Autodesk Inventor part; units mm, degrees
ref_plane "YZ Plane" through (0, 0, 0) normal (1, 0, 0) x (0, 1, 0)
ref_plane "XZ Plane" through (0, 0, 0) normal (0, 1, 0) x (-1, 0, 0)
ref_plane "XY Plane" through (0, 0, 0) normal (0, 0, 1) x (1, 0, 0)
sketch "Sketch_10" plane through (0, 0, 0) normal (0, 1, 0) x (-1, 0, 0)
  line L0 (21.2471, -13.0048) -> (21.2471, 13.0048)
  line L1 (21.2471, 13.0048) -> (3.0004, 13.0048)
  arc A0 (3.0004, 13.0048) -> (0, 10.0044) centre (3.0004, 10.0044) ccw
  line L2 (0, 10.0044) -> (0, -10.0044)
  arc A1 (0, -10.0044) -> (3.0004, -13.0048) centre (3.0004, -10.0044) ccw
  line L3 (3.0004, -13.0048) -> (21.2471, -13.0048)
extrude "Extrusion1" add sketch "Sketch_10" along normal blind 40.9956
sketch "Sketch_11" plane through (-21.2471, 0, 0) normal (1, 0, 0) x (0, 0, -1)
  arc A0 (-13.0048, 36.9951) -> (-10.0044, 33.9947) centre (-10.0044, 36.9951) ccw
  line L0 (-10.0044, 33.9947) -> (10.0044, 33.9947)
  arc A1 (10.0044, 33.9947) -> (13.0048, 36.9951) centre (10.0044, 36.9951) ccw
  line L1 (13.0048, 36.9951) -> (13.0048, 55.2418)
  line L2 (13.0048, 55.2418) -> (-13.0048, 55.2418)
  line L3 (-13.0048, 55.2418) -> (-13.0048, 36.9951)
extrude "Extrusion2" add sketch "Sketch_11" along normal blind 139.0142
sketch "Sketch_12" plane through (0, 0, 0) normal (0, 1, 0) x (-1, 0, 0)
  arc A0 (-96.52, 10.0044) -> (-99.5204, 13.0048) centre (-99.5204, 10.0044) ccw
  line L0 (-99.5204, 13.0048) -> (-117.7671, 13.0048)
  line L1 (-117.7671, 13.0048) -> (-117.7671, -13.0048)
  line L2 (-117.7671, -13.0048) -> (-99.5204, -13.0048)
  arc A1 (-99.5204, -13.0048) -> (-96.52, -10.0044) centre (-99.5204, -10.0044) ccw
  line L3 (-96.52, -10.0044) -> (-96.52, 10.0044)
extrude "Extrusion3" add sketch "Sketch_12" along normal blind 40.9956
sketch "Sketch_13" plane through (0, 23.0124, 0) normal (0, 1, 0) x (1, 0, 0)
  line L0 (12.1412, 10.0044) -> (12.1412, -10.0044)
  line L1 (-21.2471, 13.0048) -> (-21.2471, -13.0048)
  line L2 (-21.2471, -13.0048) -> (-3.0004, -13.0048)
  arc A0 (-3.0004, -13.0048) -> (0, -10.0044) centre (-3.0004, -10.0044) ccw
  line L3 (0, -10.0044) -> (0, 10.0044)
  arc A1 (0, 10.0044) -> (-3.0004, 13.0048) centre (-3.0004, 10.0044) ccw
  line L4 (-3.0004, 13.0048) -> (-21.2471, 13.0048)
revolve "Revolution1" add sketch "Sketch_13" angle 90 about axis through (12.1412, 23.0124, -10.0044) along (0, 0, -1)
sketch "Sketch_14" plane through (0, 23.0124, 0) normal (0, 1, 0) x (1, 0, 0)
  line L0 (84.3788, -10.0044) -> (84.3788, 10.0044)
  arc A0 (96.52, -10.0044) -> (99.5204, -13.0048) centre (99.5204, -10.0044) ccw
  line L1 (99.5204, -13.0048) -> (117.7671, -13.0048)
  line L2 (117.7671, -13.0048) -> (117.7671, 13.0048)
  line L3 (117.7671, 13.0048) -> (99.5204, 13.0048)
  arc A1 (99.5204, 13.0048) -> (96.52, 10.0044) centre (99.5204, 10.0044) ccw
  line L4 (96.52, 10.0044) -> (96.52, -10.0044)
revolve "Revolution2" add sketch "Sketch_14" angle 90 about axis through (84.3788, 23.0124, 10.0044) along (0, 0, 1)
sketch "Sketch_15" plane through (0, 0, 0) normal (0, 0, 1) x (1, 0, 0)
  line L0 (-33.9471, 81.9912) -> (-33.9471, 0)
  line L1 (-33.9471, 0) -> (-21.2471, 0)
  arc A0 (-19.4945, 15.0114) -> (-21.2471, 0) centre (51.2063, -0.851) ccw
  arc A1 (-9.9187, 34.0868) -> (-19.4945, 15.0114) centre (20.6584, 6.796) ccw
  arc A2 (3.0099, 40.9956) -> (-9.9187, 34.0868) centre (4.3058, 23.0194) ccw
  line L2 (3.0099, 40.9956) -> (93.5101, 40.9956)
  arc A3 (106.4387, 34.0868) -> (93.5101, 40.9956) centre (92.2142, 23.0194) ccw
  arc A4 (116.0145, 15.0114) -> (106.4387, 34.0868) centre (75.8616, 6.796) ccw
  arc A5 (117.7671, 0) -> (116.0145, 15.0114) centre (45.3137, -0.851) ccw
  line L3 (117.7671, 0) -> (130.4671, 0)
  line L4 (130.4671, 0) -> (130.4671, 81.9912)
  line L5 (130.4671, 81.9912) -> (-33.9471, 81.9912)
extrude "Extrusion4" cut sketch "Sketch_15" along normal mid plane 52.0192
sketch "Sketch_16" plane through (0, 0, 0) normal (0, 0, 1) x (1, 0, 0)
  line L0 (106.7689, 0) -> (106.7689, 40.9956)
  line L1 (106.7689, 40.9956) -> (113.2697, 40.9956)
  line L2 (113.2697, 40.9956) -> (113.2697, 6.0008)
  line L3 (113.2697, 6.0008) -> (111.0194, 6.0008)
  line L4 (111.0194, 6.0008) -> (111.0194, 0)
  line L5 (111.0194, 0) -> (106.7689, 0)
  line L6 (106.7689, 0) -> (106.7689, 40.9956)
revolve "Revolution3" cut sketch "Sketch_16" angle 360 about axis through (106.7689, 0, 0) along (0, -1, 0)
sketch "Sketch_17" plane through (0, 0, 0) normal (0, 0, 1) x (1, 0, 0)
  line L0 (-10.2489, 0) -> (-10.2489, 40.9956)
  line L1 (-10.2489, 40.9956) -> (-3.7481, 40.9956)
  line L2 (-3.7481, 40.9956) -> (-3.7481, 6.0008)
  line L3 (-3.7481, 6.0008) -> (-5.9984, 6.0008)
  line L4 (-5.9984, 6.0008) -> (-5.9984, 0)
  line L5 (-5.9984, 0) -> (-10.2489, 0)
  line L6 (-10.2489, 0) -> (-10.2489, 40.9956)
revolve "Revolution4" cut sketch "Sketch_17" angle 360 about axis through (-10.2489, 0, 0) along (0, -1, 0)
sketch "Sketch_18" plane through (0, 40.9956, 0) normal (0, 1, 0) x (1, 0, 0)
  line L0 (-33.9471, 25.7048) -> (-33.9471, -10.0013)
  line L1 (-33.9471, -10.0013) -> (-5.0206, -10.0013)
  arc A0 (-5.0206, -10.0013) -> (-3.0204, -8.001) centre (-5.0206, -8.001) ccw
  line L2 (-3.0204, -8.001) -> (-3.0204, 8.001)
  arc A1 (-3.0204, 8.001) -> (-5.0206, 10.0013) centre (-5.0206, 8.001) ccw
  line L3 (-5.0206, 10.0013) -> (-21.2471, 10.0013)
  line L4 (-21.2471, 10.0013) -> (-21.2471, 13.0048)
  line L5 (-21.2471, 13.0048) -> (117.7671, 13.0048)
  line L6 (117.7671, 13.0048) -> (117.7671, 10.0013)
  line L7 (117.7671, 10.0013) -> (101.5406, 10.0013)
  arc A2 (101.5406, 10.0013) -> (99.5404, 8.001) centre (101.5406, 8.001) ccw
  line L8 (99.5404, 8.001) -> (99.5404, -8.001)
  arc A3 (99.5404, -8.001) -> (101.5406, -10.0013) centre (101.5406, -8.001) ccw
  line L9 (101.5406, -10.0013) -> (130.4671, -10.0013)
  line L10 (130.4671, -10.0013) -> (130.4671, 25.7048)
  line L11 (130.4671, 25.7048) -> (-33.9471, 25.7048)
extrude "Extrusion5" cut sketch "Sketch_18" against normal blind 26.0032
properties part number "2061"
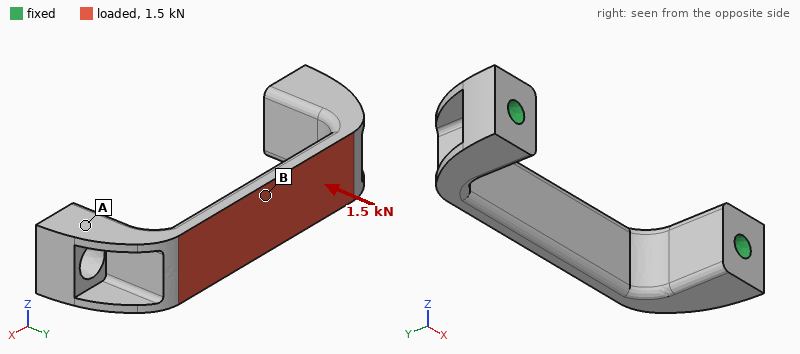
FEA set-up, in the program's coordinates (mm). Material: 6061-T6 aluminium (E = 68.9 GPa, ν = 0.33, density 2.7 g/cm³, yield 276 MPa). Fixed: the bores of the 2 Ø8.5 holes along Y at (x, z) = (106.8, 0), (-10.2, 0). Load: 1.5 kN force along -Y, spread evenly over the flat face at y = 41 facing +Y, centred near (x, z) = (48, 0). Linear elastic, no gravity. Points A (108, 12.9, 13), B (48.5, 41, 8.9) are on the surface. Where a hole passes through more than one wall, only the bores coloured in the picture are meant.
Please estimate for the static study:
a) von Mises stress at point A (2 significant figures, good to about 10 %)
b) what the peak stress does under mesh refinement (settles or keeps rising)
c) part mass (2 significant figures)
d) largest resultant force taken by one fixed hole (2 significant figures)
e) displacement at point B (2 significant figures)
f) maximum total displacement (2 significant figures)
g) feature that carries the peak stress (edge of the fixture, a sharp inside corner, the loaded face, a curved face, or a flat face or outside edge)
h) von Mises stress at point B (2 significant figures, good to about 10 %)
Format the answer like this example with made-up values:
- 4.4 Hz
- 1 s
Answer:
- 6.2 MPa
- keeps rising
- 100 g
- 990 N
- 0.10 mm
- 0.10 mm
- a sharp inside corner
- 38 MPa
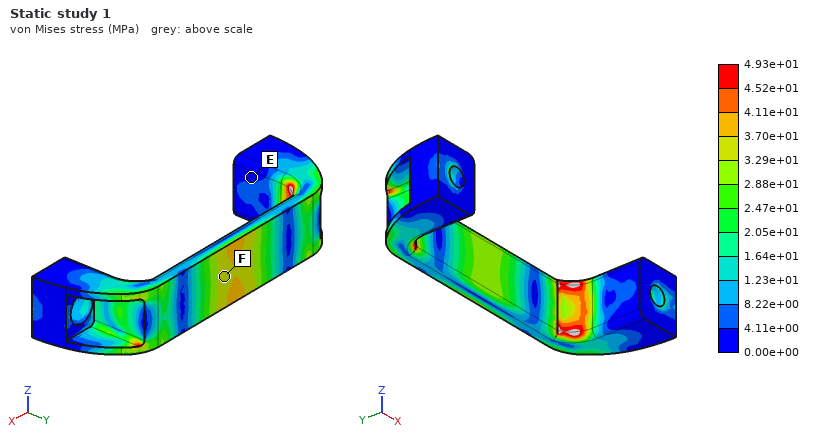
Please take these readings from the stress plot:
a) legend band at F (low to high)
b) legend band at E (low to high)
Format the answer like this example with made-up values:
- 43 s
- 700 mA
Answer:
- 3.29e+01 to 3.70e+01 MPa
- 0.00e+00 to 4.11e+00 MPa
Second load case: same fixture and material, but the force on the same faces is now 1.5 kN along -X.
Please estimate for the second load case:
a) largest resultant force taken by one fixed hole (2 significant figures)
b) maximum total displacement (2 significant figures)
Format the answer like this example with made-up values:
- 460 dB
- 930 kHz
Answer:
- 770 N
- 50 µm
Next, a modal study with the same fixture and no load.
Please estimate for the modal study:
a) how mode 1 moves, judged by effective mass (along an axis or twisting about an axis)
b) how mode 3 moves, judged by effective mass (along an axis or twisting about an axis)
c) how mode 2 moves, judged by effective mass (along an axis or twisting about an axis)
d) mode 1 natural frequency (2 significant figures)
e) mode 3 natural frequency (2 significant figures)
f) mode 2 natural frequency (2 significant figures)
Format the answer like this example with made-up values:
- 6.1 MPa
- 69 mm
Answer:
- along Z
- along X
- along Y
- 3100 Hz
- 3600 Hz
- 3300 Hz
